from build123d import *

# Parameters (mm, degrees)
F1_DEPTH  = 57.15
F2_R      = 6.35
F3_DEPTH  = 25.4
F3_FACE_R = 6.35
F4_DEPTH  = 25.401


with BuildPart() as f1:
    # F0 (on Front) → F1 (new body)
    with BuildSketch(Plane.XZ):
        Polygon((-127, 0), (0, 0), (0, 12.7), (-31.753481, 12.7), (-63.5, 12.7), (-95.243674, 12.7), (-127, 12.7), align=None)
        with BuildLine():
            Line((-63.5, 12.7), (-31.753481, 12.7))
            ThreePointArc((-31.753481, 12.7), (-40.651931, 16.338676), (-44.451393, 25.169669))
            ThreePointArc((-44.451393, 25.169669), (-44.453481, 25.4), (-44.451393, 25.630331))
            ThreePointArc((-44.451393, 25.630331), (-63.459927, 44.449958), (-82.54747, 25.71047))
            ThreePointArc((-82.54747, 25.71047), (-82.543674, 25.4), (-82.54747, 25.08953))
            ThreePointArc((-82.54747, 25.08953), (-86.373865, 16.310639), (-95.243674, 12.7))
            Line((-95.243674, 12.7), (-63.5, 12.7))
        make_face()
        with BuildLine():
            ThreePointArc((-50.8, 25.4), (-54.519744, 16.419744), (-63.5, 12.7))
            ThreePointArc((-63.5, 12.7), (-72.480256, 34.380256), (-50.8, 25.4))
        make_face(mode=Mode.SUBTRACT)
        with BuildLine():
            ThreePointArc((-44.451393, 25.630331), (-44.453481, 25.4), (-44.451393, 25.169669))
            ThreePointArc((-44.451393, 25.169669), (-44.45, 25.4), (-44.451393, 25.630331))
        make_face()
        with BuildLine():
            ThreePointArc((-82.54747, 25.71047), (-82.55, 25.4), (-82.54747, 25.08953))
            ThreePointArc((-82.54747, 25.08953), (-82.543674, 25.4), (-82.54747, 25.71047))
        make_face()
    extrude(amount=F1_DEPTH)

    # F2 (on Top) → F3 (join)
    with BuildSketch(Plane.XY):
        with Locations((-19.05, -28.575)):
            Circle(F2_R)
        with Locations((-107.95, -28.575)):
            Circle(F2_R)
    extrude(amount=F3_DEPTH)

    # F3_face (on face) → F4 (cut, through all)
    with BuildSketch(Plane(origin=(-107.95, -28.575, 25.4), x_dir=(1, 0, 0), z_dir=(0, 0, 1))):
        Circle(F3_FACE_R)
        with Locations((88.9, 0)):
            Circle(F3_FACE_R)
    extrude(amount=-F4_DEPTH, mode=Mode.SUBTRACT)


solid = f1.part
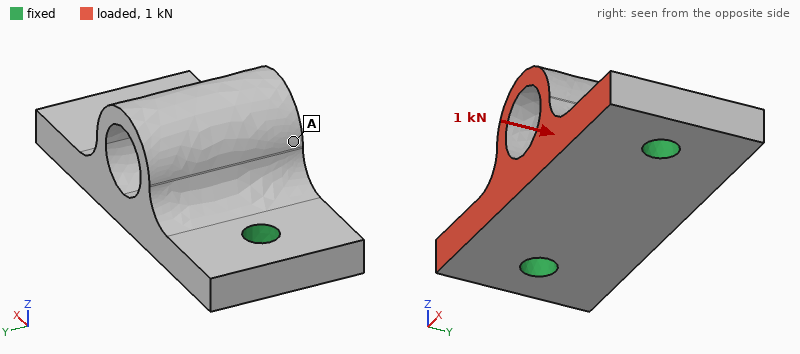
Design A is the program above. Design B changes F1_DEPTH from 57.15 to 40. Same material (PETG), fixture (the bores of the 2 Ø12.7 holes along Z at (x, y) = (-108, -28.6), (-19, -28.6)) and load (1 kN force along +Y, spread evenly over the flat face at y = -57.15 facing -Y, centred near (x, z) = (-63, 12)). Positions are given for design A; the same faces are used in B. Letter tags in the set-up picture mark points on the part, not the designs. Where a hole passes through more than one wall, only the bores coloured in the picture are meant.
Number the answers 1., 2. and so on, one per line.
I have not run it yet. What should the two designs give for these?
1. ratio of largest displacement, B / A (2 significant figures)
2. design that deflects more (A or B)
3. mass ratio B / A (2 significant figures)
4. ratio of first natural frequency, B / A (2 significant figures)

1. 1.5
2. B
3. 0.69
4. 1.0
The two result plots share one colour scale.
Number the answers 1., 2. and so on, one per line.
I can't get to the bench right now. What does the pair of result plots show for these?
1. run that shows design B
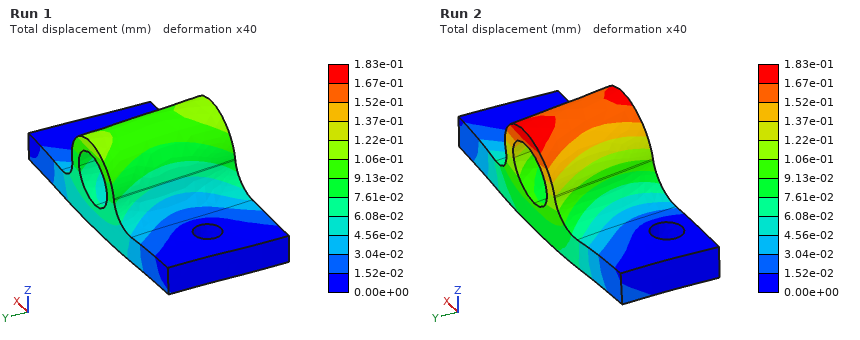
1. Run 2
